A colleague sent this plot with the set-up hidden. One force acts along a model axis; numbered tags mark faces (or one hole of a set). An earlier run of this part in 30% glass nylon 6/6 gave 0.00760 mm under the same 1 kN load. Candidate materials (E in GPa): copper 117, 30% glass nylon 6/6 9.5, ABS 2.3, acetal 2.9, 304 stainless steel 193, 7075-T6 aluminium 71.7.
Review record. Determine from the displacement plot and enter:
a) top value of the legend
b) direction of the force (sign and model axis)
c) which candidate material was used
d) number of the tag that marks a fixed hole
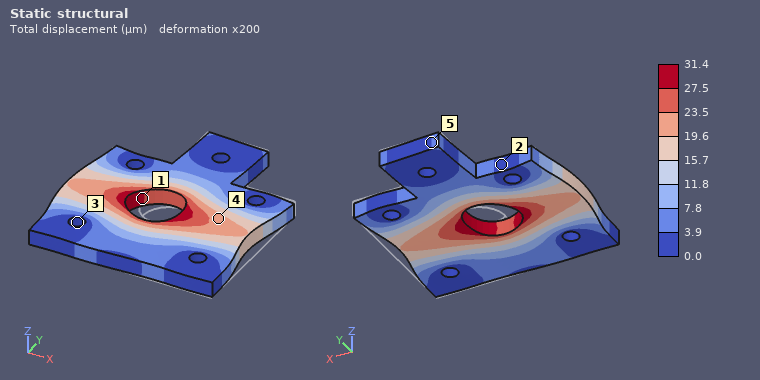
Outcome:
31.4 µm
-X
ABS
3
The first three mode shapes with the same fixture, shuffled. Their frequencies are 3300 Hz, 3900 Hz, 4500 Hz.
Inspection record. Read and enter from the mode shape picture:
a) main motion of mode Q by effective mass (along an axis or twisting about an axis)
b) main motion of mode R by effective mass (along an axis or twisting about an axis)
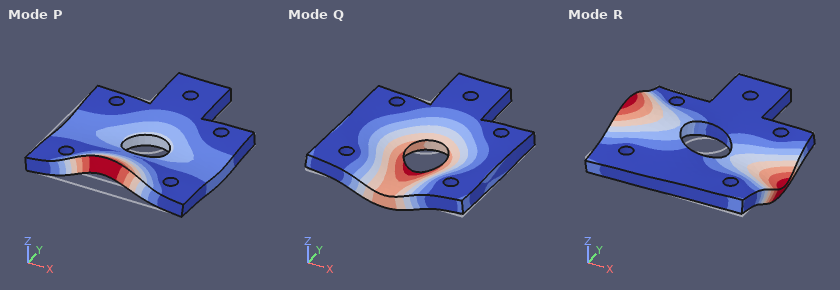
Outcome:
along Z
twisting about Y
